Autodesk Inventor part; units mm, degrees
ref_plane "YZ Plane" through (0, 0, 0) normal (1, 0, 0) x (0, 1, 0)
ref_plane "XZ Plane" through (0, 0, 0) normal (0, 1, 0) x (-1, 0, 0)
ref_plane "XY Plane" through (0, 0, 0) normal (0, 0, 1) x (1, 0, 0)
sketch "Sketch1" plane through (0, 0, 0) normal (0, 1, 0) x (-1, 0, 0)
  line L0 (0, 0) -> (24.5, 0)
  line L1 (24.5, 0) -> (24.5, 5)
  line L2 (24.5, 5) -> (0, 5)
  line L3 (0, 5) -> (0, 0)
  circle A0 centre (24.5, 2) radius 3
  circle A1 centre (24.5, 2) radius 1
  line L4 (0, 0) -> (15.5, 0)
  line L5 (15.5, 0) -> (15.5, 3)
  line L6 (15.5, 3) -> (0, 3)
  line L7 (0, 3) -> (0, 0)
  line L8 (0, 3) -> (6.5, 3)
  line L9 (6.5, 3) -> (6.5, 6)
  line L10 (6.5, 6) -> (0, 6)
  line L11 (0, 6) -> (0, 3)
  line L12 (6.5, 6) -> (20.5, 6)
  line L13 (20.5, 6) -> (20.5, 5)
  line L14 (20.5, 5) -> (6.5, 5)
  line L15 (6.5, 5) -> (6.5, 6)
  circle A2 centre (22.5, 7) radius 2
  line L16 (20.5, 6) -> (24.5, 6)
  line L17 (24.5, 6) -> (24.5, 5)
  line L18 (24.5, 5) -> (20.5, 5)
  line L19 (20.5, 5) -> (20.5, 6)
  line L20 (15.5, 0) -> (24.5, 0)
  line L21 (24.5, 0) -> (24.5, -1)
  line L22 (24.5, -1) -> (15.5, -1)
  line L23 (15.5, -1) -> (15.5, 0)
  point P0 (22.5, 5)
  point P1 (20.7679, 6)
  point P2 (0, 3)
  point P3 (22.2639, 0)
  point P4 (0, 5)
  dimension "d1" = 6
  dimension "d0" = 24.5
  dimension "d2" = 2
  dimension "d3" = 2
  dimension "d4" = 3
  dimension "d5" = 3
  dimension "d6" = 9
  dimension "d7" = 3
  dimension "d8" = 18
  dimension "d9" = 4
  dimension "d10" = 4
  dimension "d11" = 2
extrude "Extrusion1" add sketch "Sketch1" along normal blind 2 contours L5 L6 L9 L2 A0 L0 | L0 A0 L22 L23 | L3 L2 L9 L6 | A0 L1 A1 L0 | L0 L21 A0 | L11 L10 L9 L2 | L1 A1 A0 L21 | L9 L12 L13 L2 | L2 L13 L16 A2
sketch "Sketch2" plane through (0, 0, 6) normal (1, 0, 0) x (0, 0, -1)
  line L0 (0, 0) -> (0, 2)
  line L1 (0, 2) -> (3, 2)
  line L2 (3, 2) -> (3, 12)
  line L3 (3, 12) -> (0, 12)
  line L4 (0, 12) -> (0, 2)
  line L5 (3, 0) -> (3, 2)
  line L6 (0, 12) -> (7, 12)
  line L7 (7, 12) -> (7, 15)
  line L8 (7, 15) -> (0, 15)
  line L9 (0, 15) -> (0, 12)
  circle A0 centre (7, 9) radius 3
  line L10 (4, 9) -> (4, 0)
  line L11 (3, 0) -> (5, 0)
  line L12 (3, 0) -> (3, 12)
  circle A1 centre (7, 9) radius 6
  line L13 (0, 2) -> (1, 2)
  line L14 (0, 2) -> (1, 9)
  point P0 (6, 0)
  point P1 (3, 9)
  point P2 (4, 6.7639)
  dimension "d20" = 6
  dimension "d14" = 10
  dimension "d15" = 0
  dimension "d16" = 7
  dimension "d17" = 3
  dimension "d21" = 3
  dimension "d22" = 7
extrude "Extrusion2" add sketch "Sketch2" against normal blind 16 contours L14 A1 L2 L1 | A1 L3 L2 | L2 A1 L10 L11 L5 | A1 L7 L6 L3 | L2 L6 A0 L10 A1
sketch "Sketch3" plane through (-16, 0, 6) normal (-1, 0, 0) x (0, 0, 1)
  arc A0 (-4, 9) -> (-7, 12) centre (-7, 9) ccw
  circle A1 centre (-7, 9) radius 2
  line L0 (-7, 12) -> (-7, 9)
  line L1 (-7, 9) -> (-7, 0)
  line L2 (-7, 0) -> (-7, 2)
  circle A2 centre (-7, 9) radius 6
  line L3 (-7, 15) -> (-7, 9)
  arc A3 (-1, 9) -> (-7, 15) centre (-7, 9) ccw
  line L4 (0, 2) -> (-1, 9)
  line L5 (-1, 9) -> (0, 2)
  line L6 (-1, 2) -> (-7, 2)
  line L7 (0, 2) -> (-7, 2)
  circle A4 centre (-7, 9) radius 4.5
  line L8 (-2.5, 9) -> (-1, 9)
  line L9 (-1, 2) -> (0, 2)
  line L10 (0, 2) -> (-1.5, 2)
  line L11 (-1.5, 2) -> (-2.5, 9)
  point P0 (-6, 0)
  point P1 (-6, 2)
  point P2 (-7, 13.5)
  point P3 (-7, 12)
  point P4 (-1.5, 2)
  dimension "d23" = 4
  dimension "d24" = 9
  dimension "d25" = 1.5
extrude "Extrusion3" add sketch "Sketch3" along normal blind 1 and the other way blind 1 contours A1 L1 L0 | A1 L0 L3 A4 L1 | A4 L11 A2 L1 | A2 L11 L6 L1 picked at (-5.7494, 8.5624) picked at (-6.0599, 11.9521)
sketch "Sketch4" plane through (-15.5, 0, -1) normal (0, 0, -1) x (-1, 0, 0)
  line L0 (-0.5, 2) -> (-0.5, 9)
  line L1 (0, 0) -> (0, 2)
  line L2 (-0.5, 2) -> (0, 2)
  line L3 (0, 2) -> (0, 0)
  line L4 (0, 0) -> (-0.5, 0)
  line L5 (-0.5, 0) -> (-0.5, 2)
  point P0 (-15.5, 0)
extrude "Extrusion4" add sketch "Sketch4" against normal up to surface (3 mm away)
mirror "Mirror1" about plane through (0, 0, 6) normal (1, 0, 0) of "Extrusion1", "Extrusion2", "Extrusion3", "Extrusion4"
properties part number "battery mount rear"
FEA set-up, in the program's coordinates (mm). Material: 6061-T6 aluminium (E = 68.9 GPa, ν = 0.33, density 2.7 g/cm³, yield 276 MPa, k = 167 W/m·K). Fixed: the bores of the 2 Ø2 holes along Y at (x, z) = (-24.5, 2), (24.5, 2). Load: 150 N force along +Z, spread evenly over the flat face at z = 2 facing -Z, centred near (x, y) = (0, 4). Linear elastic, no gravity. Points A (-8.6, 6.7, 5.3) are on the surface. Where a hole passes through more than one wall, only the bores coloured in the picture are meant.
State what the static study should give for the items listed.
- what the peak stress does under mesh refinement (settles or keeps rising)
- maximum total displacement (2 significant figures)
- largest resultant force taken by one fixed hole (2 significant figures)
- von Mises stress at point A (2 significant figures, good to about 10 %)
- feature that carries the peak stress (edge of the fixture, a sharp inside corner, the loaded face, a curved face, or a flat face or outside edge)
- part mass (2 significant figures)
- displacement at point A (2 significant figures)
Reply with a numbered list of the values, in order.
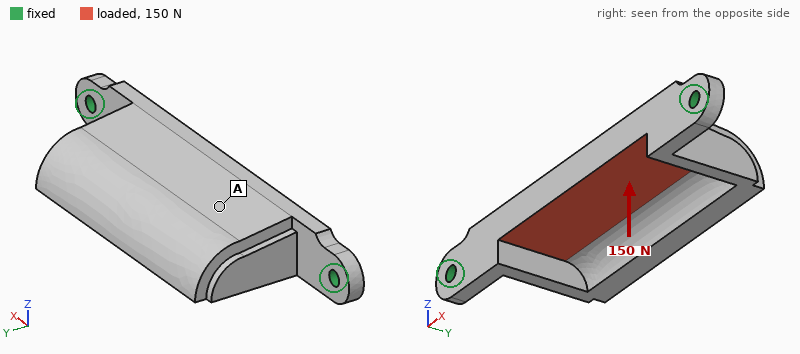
1. keeps rising
2. 90 µm
3. 130 N
4. 11 MPa
5. edge of the fixture
6. 5.8 g
7. 49 µm
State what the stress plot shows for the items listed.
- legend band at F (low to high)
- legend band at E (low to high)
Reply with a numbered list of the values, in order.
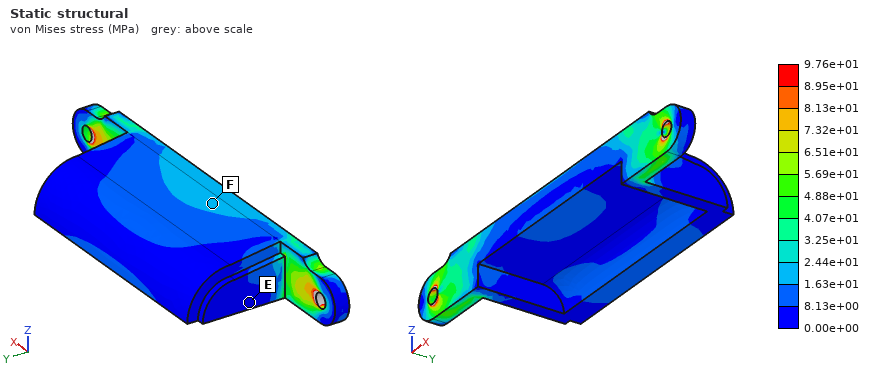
1. 1.63e+01 to 2.44e+01 MPa
2. 0.00e+00 to 8.13e+00 MPa
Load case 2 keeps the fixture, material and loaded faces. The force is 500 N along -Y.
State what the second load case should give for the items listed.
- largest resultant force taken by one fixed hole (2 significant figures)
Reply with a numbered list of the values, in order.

1. 320 N
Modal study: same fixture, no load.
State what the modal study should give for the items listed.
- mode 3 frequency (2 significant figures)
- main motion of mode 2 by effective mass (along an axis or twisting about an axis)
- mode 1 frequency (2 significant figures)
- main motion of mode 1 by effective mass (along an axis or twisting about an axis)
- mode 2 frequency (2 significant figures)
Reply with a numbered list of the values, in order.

1. 9600 Hz
2. along Y
3. 2700 Hz
4. along Z
5. 6600 Hz
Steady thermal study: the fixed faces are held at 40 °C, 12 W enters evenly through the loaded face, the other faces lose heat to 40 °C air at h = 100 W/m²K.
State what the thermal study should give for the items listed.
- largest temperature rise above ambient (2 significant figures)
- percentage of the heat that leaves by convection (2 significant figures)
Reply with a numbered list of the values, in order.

1. 26 K
2. 26 %
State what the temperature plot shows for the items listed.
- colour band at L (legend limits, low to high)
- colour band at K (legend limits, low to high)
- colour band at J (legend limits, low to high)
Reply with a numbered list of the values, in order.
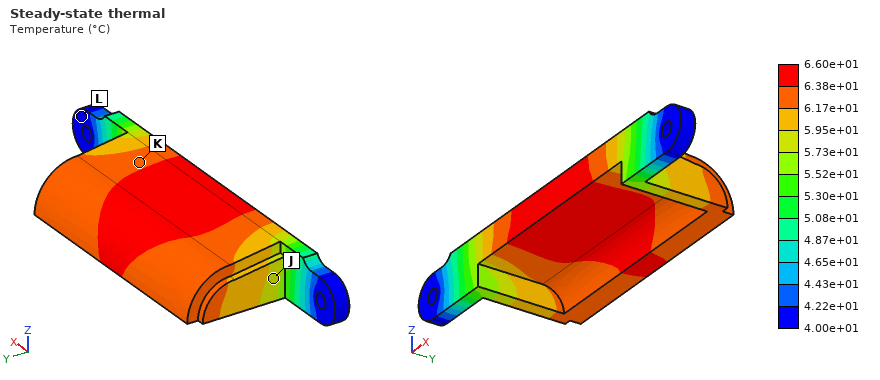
1. 4.00e+01 to 4.22e+01 °C
2. 6.17e+01 to 6.38e+01 °C
3. 5.73e+01 to 5.95e+01 °C
